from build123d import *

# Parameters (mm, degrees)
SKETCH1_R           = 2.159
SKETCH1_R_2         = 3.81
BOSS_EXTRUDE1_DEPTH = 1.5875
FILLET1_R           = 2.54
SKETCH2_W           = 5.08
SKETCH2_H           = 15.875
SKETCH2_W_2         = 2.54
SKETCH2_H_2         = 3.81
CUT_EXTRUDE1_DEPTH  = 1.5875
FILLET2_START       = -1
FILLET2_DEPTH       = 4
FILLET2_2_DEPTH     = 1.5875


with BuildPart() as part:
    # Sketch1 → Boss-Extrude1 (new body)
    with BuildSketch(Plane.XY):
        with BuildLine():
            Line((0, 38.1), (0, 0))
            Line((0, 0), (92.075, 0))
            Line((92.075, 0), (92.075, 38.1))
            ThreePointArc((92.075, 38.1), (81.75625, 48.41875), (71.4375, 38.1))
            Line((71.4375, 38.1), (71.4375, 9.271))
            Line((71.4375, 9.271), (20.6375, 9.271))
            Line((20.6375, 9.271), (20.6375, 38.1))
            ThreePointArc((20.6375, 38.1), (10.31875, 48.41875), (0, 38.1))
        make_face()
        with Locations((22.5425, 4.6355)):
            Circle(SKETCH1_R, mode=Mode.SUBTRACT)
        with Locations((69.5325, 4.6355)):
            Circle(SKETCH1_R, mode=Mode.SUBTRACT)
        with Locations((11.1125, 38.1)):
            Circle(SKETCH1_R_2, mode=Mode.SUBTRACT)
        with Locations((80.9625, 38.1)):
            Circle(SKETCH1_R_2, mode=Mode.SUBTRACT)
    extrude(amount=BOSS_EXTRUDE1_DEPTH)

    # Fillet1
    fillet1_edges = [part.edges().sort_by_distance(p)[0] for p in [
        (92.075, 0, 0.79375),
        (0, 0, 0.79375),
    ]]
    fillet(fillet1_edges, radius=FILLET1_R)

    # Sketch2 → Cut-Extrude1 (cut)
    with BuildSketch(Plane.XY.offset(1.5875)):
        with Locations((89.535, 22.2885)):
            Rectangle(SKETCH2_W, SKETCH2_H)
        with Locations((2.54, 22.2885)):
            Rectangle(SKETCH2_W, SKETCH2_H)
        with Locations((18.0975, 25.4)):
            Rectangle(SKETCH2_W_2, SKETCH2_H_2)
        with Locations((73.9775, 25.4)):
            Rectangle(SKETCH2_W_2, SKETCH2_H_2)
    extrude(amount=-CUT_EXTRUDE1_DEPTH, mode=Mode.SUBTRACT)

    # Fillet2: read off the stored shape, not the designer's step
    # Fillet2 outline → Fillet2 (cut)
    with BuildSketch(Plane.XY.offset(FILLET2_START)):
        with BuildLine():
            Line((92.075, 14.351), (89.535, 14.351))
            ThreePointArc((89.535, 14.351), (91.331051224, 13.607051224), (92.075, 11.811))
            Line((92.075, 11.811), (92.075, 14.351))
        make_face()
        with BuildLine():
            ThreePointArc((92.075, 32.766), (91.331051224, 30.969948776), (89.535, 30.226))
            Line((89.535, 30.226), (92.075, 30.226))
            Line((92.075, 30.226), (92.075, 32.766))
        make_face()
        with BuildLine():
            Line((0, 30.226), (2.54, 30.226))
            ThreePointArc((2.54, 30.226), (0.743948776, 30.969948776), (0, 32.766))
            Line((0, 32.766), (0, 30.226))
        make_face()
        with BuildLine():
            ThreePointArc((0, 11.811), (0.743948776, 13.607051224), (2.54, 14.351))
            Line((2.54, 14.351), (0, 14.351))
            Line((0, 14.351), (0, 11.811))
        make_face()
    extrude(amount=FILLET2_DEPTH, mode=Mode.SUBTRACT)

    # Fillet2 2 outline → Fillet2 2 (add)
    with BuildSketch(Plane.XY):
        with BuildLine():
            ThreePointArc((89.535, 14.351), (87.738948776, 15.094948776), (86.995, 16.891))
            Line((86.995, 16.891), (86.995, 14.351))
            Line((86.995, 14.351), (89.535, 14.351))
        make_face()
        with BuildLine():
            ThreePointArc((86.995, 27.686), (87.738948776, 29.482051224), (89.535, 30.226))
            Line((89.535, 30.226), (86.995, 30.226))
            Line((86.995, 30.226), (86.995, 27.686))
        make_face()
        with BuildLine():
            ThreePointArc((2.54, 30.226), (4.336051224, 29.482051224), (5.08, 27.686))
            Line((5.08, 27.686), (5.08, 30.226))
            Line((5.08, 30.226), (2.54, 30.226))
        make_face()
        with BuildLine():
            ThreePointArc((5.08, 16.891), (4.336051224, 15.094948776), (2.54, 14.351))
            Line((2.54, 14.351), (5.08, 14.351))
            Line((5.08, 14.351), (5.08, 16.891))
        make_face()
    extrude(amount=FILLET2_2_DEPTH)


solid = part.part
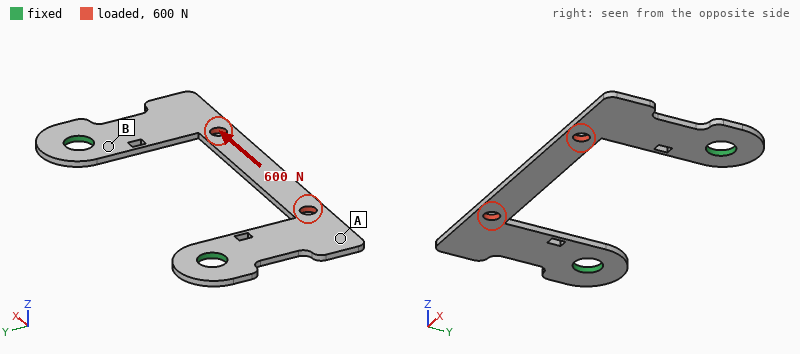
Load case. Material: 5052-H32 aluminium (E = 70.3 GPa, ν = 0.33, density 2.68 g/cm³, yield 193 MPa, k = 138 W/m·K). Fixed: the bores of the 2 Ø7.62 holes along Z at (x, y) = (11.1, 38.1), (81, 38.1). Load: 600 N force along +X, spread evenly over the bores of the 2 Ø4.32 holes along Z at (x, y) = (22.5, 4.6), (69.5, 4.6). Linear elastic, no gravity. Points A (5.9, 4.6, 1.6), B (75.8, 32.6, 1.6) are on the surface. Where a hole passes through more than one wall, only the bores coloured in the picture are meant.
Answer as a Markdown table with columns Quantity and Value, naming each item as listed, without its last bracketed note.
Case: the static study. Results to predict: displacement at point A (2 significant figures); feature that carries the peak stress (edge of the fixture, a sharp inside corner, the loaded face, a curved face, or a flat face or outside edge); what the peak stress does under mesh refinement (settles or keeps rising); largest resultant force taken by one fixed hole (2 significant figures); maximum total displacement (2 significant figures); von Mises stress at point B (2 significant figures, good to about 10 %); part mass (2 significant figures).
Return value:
| Quantity | Value |
|---|---|
| displacement at point A | 0.086 mm |
| feature that carries the peak stress | a sharp inside corner |
| what the peak stress does under mesh refinement | keeps rising |
| largest resultant force taken by one fixed hole | 310 N |
| maximum total displacement | 0.10 mm |
| von Mises stress at point B | 43 MPa |
| part mass | 8.8 g |
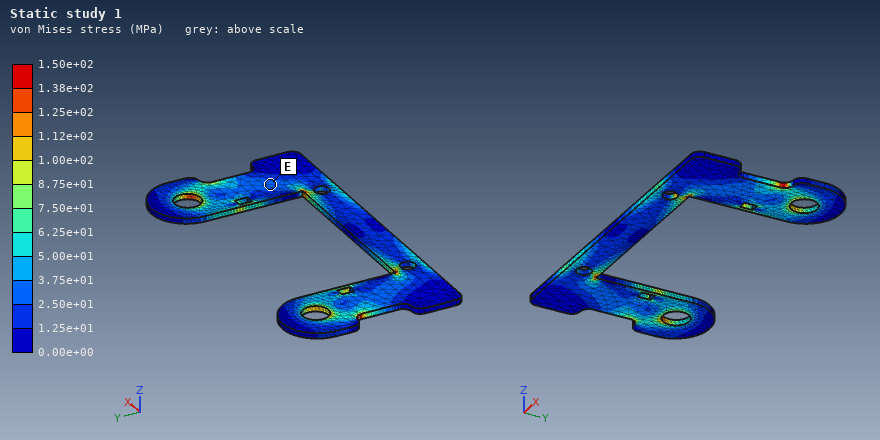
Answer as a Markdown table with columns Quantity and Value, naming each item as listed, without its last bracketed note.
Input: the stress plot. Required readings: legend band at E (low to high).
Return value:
| Quantity | Value |
|---|---|
| legend band at E | 2.50e+01 to 3.75e+01 MPa |
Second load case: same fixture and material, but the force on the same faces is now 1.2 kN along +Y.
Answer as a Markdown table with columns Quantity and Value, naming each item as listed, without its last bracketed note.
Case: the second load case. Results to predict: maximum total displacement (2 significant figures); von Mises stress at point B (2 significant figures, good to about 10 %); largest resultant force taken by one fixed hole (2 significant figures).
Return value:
| Quantity | Value |
|---|---|
| maximum total displacement | 66 µm |
| von Mises stress at point B | 22 MPa |
| largest resultant force taken by one fixed hole | 640 N |
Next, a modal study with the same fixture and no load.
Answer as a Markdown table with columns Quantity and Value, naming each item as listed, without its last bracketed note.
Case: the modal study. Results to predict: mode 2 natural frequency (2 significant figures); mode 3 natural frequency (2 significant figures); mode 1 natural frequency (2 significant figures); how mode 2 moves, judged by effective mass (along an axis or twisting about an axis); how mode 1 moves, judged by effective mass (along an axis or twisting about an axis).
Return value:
| Quantity | Value |
|---|---|
| mode 2 natural frequency | 1100 Hz |
| mode 3 natural frequency | 1700 Hz |
| mode 1 natural frequency | 660 Hz |
| how mode 2 moves, judged by effective mass | twisting about Y |
| how mode 1 moves, judged by effective mass | along Z |
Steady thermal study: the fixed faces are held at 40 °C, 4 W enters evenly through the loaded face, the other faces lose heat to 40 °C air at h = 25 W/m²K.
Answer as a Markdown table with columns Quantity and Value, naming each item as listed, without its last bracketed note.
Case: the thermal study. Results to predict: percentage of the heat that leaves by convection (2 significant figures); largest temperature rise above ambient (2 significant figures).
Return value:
| Quantity | Value |
|---|---|
| percentage of the heat that leaves by convection | 27 % |
| largest temperature rise above ambient | 20 K |
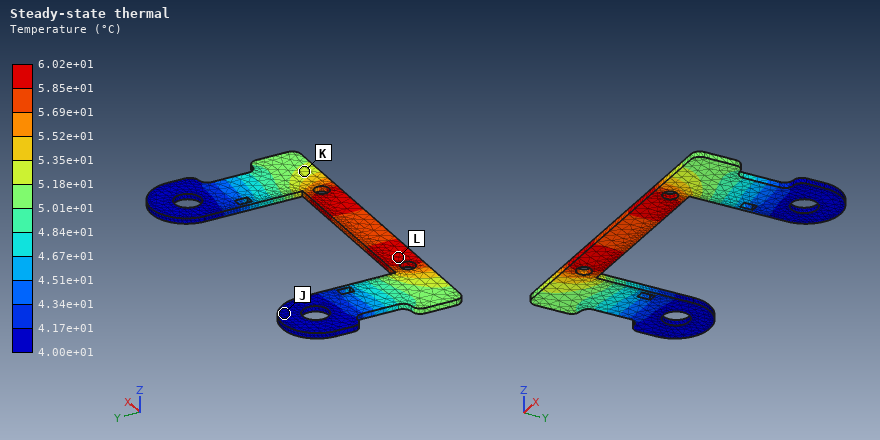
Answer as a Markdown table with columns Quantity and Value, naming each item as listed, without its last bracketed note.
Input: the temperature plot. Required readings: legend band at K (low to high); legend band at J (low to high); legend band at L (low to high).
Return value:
| Quantity | Value |
|---|---|
| legend band at K | 5.18e+01 to 5.35e+01 °C |
| legend band at J | 4.00e+01 to 4.17e+01 °C |
| legend band at L | 5.85e+01 to 6.02e+01 °C |
